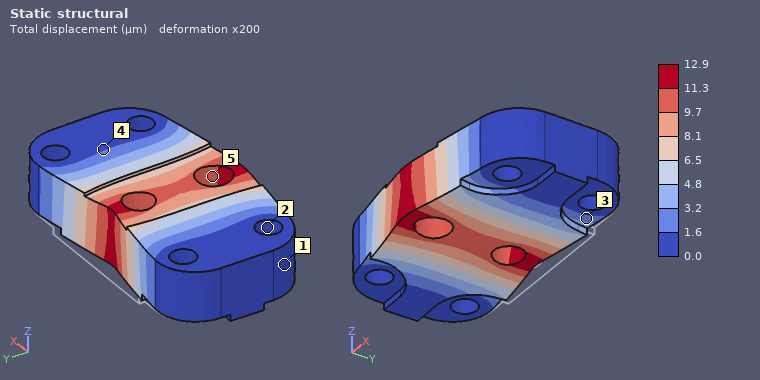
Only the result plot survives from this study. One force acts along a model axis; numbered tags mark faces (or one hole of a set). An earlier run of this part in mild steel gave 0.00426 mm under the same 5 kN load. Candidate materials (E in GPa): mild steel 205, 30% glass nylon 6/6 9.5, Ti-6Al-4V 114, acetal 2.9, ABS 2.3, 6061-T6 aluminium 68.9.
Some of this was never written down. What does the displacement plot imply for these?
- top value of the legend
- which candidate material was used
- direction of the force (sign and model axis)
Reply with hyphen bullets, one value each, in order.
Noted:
- 12.9 µm
- 6061-T6 aluminium
- -Y
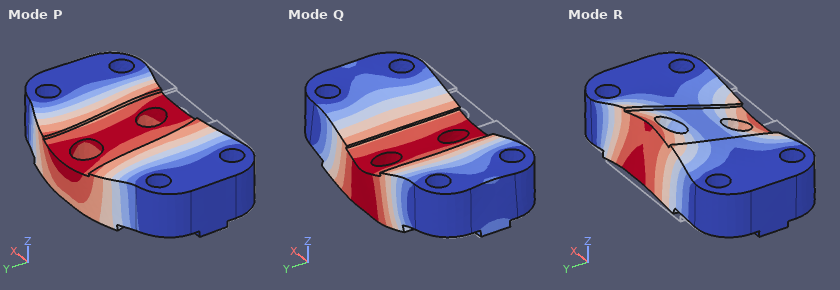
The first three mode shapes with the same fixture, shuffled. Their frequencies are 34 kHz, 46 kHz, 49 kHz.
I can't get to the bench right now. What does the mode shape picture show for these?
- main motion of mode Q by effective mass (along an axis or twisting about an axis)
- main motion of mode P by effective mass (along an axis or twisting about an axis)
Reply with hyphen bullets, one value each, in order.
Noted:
- along Z
- along Y
